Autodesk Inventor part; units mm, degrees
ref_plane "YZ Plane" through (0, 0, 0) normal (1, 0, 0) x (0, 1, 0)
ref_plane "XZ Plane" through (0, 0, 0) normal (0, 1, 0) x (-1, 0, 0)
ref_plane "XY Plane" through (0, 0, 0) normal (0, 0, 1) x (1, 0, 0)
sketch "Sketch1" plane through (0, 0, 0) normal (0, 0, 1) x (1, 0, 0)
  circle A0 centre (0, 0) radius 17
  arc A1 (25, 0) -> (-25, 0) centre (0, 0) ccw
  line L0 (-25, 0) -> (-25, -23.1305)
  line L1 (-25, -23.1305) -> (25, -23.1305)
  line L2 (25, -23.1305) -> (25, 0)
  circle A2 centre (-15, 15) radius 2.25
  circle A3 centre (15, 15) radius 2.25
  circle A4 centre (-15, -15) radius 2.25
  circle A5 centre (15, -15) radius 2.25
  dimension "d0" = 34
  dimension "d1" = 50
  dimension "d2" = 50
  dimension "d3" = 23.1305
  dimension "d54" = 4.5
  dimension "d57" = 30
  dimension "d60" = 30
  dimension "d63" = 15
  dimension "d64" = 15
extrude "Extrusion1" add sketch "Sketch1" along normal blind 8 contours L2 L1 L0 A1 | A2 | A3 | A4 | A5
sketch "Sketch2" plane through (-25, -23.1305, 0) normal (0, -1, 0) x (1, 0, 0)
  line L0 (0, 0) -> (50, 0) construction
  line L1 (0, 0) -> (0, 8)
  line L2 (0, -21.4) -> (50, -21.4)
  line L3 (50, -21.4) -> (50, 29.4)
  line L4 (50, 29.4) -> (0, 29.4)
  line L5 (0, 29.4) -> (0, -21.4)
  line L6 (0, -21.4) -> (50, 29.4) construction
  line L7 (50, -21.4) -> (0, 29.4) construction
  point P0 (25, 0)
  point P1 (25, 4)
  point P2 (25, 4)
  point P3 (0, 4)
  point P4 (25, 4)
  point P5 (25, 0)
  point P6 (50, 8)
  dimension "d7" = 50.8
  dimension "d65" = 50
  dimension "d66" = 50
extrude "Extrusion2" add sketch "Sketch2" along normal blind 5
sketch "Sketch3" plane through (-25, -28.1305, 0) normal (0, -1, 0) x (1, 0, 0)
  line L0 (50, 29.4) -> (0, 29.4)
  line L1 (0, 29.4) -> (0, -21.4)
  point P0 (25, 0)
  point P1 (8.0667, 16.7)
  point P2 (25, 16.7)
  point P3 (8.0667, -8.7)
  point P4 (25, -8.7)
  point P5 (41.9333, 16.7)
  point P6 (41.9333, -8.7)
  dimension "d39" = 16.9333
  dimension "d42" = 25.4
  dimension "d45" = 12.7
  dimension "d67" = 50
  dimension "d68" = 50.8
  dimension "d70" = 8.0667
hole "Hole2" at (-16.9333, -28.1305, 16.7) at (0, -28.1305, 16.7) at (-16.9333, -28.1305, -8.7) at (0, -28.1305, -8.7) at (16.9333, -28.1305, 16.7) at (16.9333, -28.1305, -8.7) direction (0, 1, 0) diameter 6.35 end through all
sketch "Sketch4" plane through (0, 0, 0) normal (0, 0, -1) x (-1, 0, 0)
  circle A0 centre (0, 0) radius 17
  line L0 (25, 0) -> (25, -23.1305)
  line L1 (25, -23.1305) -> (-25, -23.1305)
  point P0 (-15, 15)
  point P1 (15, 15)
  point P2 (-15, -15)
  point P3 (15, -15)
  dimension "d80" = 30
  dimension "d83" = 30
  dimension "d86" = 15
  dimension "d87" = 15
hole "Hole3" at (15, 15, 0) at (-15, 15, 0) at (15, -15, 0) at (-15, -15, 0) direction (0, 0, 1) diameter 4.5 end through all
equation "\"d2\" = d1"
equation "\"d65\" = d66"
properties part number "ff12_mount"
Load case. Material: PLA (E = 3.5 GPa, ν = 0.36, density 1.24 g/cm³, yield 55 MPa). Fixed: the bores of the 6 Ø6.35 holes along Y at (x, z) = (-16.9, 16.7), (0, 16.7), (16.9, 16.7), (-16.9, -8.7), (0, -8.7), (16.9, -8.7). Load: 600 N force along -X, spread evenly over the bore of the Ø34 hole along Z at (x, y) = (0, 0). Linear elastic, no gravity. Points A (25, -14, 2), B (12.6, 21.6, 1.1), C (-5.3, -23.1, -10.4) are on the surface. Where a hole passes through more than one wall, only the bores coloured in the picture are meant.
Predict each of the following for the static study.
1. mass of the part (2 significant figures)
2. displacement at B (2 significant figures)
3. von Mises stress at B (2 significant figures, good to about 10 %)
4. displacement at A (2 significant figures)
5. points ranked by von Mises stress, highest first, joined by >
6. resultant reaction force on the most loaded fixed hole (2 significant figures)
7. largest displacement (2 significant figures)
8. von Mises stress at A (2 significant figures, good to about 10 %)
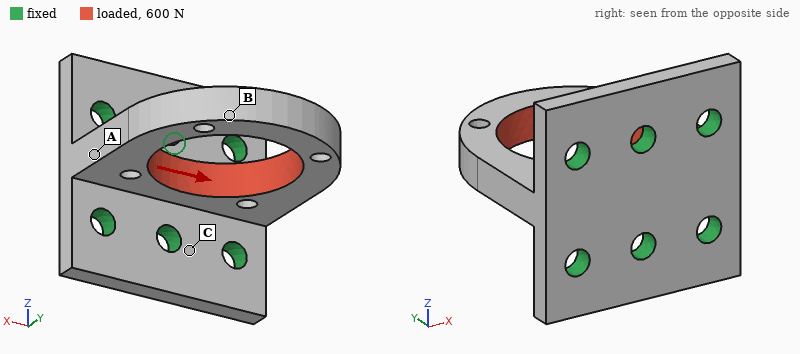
26 g
0.53 mm
8.3 MPa
0.13 mm
A > B > C
240 N
0.53 mm
13 MPa
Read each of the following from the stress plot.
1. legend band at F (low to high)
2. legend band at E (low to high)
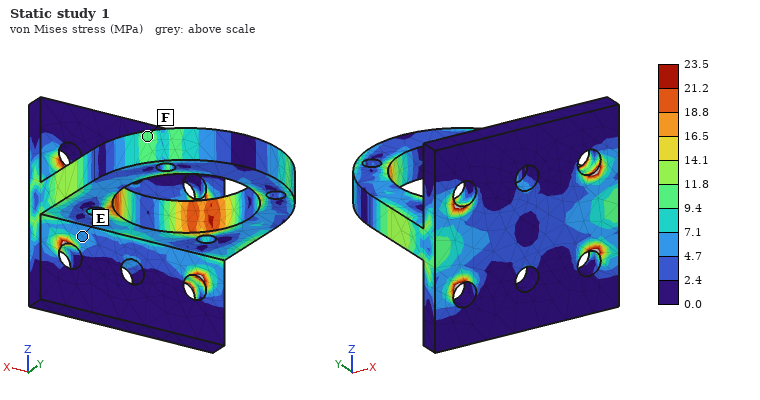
9.4 to 11.8 MPa
4.7 to 7.1 MPa
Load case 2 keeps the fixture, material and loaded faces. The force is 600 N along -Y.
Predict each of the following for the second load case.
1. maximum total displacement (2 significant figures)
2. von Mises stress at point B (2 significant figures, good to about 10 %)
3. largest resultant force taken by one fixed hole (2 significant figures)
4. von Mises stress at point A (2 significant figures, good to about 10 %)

0.12 mm
3.2 MPa
130 N
2.5 MPa
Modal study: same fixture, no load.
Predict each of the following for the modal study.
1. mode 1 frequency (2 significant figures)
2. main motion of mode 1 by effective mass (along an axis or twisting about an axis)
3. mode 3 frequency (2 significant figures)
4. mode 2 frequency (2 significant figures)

840 Hz
along Z
2000 Hz
1900 Hz
